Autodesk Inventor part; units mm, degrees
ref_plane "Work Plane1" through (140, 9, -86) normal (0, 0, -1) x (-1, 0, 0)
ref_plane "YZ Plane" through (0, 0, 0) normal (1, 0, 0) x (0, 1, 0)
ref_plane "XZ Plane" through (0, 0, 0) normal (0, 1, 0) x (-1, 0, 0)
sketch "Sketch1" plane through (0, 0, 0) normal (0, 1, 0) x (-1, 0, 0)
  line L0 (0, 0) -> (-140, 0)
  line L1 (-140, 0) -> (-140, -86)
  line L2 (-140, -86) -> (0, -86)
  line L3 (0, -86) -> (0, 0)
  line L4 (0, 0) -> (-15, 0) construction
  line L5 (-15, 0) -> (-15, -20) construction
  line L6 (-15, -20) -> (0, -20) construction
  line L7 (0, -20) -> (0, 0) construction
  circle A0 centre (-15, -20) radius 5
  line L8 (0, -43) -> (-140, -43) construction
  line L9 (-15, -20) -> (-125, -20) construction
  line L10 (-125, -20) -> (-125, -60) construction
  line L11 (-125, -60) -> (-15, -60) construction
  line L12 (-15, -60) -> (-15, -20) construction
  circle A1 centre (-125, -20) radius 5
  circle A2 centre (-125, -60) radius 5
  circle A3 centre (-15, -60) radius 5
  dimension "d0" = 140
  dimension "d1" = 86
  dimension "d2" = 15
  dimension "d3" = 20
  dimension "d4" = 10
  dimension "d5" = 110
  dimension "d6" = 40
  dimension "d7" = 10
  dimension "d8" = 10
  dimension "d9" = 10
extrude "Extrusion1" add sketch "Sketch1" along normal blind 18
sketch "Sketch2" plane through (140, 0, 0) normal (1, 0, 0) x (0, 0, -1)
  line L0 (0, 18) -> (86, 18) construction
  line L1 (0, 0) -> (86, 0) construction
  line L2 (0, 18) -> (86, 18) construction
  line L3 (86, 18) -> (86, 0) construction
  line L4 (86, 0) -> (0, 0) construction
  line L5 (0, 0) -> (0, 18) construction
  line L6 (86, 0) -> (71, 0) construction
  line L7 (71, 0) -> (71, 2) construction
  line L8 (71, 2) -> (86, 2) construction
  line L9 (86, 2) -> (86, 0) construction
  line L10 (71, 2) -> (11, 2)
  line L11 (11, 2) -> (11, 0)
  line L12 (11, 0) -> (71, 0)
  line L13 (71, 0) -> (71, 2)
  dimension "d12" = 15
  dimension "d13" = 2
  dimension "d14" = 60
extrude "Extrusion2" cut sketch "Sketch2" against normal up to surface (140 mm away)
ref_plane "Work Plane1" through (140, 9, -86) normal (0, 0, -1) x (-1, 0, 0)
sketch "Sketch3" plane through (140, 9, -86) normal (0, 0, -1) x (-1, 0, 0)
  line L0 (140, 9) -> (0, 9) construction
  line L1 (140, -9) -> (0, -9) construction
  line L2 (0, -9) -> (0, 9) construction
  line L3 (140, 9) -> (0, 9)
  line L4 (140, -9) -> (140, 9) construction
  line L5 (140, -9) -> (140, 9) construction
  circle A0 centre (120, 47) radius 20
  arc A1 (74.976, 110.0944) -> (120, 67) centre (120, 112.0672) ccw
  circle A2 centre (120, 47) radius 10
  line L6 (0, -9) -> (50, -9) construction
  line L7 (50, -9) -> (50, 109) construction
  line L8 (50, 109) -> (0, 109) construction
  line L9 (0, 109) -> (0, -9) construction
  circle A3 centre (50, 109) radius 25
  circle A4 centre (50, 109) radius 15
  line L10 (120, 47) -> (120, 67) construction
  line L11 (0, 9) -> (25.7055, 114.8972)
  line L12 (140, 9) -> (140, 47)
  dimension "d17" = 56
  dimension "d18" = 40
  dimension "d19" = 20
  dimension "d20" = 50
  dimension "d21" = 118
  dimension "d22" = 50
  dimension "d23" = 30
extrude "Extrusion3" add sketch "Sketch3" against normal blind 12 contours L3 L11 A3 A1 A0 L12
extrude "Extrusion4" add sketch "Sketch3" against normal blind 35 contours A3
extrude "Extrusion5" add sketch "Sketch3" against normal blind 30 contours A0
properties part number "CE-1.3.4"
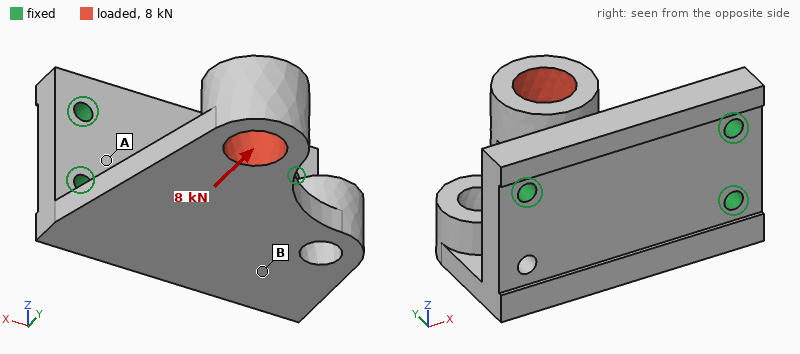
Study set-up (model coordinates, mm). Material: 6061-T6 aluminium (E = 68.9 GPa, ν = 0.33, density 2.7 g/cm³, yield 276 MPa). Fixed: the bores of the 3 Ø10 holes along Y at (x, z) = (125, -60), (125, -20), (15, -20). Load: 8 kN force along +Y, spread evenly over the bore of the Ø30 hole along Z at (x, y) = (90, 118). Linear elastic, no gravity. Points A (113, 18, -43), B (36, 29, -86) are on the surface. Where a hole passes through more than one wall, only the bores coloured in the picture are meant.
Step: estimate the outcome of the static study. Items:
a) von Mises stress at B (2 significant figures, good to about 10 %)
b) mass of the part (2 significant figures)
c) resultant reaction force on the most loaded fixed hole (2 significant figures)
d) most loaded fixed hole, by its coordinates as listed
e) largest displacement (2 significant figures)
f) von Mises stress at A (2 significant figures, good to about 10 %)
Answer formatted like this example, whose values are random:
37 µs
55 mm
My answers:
22 MPa
990 g
6.4 kN
(125, -60)
0.63 mm
11 MPa
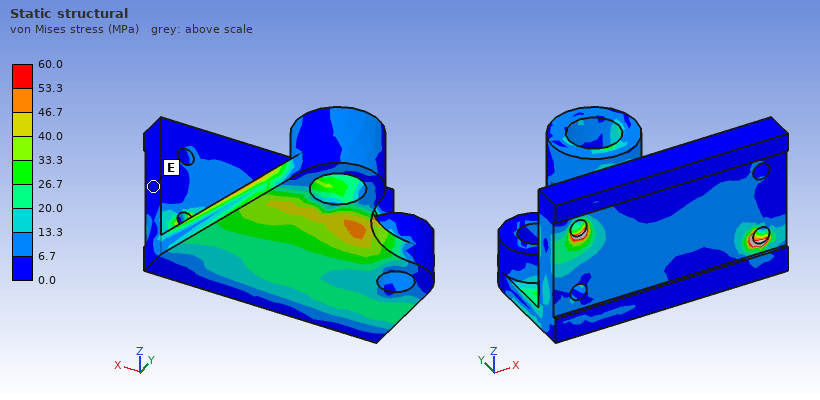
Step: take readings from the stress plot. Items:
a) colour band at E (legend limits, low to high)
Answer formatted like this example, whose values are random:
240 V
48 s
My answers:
0.0 to 6.7 MPa
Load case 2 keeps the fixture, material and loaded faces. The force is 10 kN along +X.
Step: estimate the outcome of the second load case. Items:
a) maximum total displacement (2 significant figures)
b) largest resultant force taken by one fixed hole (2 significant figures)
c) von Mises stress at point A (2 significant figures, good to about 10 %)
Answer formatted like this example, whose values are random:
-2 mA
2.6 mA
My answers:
0.97 mm
9.2 kN
34 MPa
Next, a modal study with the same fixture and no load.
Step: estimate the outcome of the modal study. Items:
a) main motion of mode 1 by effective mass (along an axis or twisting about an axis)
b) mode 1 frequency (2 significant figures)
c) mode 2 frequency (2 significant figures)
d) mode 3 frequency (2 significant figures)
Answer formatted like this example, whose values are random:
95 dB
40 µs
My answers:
along Z
590 Hz
1200 Hz
2300 Hz
